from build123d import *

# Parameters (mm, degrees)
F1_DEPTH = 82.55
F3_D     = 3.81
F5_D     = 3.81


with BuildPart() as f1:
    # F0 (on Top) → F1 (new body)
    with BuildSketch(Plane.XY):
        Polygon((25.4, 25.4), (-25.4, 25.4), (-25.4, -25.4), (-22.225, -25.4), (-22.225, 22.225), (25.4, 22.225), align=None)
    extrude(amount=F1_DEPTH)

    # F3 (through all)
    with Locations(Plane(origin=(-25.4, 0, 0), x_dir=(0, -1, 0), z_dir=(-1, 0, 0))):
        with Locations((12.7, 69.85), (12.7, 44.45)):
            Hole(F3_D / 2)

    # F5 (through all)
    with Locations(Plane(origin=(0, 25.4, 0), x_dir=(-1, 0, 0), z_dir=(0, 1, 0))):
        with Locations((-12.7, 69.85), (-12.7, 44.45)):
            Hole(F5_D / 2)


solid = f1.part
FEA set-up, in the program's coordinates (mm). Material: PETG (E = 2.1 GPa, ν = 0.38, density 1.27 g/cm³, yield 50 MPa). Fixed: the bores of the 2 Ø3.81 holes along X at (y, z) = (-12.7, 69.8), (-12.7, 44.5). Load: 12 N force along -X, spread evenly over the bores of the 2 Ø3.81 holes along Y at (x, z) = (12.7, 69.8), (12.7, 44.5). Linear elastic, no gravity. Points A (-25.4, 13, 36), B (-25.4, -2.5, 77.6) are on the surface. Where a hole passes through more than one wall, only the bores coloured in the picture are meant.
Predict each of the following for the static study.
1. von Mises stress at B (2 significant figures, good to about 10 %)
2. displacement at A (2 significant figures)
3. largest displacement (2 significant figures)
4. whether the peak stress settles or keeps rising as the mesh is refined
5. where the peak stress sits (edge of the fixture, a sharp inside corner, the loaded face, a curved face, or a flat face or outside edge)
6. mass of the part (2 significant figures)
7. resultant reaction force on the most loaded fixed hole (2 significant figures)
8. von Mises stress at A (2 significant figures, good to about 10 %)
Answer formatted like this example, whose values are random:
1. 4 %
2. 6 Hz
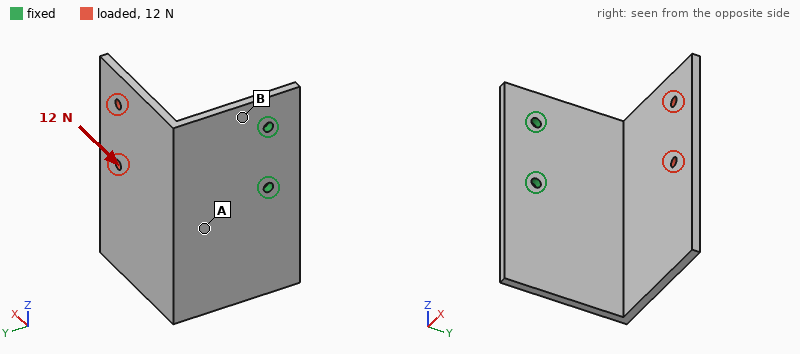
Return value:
1. 3.0 MPa
2. 0.33 mm
3. 1.2 mm
4. keeps rising
5. edge of the fixture
6. 33 g
7. 6.2 N
8. 0.96 MPa
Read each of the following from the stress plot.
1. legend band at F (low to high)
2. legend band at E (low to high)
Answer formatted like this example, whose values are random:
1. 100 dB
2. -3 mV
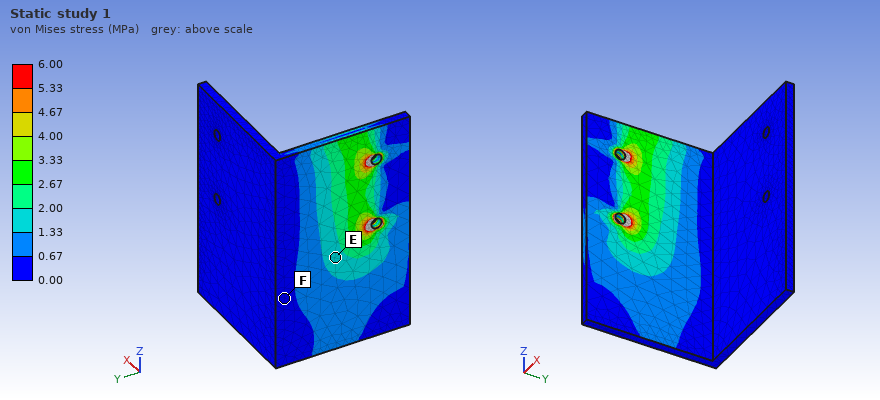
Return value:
1. 0.00 to 0.67 MPa
2. 1.33 to 2.00 MPa
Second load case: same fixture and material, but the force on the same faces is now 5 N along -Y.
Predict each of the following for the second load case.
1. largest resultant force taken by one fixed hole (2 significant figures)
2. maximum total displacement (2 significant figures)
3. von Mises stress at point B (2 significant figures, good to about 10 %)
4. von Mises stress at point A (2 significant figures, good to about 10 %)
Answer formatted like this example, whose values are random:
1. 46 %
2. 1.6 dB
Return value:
1. 2.6 N
2. 1.1 mm
3. 1.5 MPa
4. 1.1 MPa
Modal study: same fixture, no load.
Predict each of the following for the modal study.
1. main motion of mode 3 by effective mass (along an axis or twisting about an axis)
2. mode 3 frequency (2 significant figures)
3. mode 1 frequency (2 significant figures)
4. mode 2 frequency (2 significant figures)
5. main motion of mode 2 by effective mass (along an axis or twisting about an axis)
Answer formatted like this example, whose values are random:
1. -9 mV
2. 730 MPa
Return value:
1. along X
2. 310 Hz
3. 110 Hz
4. 160 Hz
5. along Z
